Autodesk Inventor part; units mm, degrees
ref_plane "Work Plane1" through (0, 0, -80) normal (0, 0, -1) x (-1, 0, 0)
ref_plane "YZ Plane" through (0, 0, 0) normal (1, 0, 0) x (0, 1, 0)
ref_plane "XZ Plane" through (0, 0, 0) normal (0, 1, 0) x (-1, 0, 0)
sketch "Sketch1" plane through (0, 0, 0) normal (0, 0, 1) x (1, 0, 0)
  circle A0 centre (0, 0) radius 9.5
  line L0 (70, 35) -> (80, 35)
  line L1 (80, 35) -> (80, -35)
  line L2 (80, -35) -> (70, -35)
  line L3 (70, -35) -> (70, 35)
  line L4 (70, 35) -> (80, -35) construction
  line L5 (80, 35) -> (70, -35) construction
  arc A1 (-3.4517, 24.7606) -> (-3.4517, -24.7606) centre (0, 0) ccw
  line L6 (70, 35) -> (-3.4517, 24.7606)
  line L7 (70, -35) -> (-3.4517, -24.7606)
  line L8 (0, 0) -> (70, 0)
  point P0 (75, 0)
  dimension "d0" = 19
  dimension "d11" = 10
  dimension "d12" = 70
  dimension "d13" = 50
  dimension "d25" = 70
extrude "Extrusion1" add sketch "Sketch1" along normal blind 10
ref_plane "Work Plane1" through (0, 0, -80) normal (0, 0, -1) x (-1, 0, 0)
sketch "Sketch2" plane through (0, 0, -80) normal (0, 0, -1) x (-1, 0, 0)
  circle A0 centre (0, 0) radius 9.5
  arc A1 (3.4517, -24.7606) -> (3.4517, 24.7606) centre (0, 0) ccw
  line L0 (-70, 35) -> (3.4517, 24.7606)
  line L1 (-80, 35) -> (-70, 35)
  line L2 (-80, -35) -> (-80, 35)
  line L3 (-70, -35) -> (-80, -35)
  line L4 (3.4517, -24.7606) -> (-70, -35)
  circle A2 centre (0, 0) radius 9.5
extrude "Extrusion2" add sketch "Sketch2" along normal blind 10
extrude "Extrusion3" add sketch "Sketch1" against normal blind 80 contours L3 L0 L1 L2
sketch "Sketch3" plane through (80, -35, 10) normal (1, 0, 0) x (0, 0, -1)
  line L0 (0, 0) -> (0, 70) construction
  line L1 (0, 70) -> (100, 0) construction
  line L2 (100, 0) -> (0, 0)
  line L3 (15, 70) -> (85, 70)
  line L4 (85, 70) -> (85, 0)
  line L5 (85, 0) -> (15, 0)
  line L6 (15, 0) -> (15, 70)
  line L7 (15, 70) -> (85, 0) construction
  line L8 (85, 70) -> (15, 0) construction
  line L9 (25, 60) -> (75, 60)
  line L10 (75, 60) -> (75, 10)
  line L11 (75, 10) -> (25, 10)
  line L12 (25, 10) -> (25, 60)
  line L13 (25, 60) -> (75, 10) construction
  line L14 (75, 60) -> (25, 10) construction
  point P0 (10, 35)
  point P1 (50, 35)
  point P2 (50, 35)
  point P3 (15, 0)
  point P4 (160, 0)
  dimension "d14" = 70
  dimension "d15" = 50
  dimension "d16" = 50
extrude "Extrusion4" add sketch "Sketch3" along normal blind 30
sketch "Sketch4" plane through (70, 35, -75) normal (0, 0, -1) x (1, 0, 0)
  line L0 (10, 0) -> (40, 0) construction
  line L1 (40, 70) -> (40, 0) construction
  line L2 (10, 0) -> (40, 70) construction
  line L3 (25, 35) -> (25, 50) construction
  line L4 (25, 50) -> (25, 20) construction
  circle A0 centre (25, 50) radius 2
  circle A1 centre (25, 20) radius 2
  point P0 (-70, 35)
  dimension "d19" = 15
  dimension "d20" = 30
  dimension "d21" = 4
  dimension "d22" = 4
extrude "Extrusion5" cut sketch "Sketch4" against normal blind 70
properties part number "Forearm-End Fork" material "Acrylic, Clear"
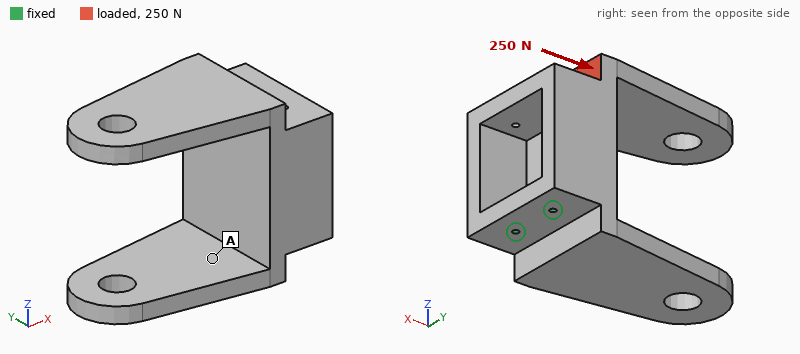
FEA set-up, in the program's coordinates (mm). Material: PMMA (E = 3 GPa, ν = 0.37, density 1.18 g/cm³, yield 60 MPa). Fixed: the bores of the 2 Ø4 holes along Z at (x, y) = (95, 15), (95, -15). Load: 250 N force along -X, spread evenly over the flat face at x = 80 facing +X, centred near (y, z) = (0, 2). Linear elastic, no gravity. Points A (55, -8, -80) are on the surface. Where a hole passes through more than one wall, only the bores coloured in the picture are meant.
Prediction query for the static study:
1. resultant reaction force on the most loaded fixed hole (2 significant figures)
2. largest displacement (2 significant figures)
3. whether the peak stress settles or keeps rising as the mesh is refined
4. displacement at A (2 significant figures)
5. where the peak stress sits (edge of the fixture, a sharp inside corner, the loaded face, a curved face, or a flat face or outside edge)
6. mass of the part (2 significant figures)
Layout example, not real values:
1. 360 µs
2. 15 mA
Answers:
1. 130 N
2. 2.0 mm
3. keeps rising
4. 0.47 mm
5. edge of the fixture
6. 280 g
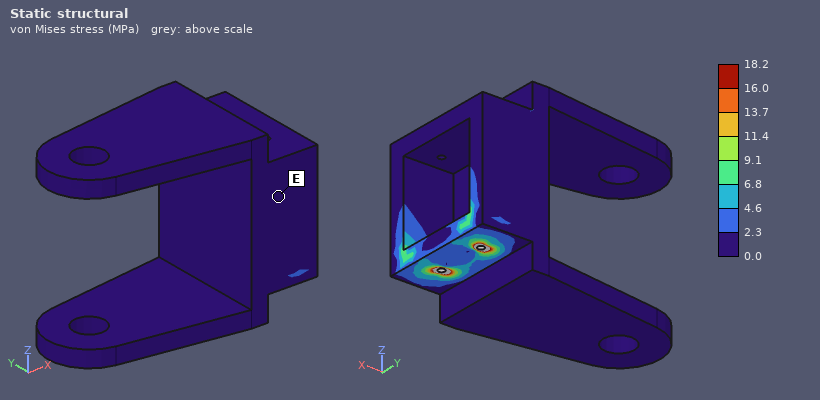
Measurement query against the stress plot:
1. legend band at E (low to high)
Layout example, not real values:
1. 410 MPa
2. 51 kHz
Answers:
1. 0.0 to 2.3 MPa
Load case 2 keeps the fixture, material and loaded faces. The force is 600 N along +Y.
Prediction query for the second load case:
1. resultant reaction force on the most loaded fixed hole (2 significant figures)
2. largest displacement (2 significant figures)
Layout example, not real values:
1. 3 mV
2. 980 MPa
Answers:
1. 1.2 kN
2. 0.88 mm
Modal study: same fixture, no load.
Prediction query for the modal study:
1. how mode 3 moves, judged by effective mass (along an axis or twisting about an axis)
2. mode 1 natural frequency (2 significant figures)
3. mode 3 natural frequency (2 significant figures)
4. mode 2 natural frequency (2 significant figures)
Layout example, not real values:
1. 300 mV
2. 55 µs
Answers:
1. along X
2. 160 Hz
3. 420 Hz
4. 280 Hz
